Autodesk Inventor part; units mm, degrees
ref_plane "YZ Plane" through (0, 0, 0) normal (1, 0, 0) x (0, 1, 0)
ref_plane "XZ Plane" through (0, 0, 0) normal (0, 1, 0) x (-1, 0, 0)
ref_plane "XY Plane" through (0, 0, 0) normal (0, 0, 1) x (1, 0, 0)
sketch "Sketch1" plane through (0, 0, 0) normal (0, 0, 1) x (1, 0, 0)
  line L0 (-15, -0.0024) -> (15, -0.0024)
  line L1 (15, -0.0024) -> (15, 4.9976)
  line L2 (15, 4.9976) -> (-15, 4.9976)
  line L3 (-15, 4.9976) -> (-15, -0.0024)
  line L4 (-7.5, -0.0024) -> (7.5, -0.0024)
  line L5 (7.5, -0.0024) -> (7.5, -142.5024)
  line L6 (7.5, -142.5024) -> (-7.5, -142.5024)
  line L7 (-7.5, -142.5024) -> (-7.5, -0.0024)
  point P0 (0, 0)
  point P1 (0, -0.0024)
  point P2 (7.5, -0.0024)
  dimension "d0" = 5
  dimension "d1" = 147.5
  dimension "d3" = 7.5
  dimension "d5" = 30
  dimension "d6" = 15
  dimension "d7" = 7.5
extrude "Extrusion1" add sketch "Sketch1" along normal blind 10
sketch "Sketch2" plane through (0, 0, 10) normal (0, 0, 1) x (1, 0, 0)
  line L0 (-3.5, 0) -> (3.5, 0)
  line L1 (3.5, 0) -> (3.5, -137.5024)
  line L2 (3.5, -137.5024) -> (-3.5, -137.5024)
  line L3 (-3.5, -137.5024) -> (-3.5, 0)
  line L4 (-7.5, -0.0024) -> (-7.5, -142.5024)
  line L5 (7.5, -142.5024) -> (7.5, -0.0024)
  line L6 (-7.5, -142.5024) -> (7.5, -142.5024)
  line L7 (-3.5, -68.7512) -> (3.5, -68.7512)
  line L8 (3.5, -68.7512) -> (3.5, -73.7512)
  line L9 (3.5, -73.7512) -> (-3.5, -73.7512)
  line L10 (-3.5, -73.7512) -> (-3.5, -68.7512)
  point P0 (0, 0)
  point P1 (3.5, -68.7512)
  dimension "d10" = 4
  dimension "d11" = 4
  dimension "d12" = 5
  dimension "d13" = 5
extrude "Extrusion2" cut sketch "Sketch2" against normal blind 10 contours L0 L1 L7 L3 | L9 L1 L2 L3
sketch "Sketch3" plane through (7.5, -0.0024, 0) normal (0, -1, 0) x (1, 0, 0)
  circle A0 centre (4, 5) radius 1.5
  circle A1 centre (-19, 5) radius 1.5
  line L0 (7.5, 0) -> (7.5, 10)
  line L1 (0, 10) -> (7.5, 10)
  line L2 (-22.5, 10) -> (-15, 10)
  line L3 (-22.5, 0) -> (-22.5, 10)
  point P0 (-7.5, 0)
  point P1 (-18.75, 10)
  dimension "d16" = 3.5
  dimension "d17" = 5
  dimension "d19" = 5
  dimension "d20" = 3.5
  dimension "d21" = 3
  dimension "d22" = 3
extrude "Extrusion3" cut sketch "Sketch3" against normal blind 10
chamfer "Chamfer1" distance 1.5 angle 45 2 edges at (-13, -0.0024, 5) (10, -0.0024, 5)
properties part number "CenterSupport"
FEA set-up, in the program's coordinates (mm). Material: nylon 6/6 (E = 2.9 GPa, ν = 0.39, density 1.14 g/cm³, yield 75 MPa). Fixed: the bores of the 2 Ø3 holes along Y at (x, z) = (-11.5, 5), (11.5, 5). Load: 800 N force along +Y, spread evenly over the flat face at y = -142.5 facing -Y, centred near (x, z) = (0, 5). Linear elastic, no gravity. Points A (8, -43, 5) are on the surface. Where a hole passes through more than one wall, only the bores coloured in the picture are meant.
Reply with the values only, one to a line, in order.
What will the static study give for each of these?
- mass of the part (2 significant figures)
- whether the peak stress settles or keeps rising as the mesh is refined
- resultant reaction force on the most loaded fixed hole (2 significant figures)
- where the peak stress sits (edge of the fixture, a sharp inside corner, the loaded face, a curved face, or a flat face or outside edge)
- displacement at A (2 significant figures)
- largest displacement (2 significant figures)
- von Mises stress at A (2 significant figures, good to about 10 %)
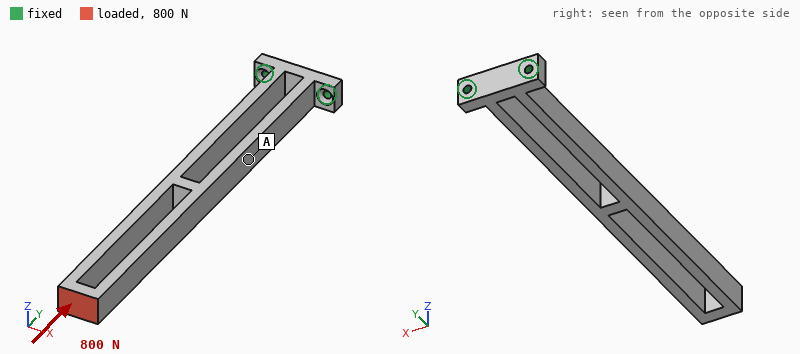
15 g
keeps rising
430 N
edge of the fixture
0.29 mm
0.63 mm
10 MPa
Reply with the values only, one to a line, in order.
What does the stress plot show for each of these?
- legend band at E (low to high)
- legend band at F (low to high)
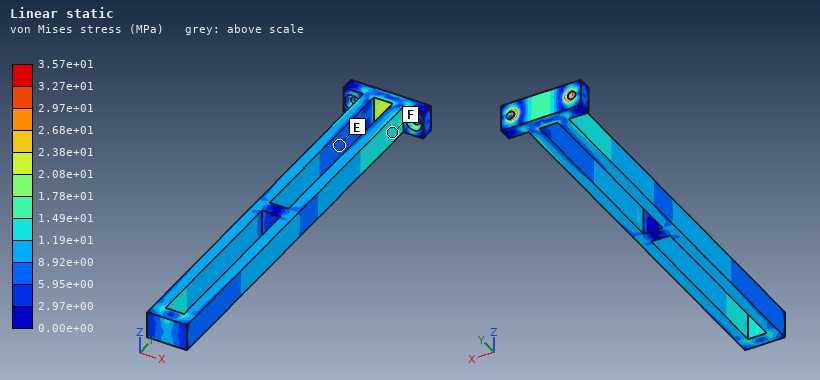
5.95e+00 to 8.92e+00 MPa
1.19e+01 to 1.49e+01 MPa
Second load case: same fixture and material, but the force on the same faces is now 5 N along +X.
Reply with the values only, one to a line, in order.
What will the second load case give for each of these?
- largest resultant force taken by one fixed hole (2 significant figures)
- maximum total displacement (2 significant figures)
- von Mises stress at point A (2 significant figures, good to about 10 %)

37 N
1.7 mm
0.85 MPa
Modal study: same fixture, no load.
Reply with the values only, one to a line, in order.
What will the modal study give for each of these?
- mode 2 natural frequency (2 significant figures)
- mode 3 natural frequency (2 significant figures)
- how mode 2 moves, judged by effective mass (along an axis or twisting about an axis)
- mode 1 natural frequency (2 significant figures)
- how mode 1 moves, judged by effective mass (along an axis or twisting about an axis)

130 Hz
410 Hz
along X
94 Hz
along Z
